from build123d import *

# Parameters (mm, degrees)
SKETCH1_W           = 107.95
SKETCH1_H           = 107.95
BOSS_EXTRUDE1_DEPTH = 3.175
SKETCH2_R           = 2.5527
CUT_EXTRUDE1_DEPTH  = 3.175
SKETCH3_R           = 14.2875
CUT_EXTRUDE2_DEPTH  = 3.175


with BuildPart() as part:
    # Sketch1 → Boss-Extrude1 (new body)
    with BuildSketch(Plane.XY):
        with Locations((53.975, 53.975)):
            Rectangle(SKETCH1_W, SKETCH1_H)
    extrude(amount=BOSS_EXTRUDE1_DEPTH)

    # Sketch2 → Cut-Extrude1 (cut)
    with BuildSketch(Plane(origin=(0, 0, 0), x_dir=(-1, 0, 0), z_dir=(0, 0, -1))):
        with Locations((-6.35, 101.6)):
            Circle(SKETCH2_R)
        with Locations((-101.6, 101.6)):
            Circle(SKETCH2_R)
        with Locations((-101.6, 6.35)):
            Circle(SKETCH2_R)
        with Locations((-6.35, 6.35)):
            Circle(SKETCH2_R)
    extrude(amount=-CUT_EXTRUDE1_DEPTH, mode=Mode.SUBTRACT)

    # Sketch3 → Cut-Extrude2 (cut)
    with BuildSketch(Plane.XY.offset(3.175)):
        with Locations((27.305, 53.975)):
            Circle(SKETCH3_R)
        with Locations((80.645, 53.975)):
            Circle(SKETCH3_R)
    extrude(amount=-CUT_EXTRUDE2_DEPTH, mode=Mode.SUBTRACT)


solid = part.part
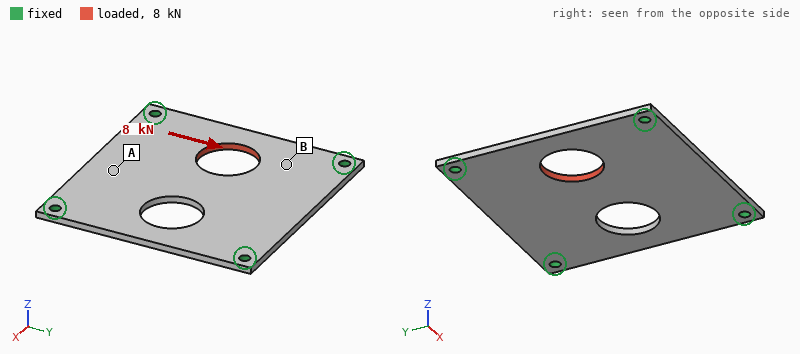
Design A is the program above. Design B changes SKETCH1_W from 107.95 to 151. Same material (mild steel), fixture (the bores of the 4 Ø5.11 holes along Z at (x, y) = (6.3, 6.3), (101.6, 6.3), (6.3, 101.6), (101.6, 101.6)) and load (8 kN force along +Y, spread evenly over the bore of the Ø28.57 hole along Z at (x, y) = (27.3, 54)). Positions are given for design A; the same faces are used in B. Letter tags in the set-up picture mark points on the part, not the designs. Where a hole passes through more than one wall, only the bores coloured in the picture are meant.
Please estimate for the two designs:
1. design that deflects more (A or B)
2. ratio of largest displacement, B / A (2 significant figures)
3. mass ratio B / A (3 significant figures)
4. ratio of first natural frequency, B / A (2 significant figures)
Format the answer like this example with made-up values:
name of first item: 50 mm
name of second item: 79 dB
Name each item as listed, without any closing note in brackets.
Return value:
design that deflects more: A
ratio of largest displacement, B / A: 0.92
mass ratio B / A: 1.45
ratio of first natural frequency, B / A: 1.1
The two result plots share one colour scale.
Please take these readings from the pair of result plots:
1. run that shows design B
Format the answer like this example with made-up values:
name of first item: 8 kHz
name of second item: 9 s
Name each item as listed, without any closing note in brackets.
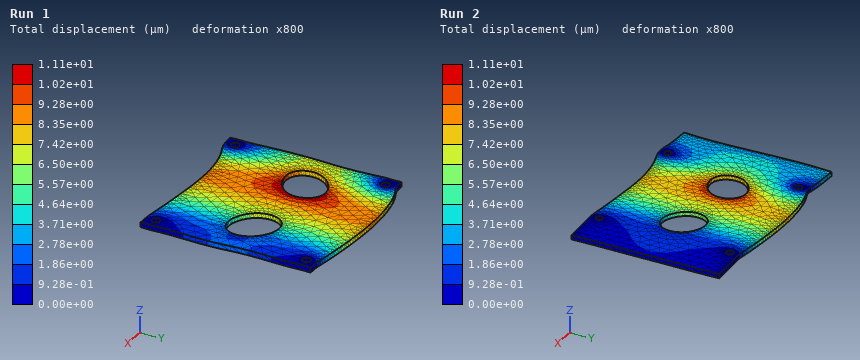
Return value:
run that shows design B: Run 2
